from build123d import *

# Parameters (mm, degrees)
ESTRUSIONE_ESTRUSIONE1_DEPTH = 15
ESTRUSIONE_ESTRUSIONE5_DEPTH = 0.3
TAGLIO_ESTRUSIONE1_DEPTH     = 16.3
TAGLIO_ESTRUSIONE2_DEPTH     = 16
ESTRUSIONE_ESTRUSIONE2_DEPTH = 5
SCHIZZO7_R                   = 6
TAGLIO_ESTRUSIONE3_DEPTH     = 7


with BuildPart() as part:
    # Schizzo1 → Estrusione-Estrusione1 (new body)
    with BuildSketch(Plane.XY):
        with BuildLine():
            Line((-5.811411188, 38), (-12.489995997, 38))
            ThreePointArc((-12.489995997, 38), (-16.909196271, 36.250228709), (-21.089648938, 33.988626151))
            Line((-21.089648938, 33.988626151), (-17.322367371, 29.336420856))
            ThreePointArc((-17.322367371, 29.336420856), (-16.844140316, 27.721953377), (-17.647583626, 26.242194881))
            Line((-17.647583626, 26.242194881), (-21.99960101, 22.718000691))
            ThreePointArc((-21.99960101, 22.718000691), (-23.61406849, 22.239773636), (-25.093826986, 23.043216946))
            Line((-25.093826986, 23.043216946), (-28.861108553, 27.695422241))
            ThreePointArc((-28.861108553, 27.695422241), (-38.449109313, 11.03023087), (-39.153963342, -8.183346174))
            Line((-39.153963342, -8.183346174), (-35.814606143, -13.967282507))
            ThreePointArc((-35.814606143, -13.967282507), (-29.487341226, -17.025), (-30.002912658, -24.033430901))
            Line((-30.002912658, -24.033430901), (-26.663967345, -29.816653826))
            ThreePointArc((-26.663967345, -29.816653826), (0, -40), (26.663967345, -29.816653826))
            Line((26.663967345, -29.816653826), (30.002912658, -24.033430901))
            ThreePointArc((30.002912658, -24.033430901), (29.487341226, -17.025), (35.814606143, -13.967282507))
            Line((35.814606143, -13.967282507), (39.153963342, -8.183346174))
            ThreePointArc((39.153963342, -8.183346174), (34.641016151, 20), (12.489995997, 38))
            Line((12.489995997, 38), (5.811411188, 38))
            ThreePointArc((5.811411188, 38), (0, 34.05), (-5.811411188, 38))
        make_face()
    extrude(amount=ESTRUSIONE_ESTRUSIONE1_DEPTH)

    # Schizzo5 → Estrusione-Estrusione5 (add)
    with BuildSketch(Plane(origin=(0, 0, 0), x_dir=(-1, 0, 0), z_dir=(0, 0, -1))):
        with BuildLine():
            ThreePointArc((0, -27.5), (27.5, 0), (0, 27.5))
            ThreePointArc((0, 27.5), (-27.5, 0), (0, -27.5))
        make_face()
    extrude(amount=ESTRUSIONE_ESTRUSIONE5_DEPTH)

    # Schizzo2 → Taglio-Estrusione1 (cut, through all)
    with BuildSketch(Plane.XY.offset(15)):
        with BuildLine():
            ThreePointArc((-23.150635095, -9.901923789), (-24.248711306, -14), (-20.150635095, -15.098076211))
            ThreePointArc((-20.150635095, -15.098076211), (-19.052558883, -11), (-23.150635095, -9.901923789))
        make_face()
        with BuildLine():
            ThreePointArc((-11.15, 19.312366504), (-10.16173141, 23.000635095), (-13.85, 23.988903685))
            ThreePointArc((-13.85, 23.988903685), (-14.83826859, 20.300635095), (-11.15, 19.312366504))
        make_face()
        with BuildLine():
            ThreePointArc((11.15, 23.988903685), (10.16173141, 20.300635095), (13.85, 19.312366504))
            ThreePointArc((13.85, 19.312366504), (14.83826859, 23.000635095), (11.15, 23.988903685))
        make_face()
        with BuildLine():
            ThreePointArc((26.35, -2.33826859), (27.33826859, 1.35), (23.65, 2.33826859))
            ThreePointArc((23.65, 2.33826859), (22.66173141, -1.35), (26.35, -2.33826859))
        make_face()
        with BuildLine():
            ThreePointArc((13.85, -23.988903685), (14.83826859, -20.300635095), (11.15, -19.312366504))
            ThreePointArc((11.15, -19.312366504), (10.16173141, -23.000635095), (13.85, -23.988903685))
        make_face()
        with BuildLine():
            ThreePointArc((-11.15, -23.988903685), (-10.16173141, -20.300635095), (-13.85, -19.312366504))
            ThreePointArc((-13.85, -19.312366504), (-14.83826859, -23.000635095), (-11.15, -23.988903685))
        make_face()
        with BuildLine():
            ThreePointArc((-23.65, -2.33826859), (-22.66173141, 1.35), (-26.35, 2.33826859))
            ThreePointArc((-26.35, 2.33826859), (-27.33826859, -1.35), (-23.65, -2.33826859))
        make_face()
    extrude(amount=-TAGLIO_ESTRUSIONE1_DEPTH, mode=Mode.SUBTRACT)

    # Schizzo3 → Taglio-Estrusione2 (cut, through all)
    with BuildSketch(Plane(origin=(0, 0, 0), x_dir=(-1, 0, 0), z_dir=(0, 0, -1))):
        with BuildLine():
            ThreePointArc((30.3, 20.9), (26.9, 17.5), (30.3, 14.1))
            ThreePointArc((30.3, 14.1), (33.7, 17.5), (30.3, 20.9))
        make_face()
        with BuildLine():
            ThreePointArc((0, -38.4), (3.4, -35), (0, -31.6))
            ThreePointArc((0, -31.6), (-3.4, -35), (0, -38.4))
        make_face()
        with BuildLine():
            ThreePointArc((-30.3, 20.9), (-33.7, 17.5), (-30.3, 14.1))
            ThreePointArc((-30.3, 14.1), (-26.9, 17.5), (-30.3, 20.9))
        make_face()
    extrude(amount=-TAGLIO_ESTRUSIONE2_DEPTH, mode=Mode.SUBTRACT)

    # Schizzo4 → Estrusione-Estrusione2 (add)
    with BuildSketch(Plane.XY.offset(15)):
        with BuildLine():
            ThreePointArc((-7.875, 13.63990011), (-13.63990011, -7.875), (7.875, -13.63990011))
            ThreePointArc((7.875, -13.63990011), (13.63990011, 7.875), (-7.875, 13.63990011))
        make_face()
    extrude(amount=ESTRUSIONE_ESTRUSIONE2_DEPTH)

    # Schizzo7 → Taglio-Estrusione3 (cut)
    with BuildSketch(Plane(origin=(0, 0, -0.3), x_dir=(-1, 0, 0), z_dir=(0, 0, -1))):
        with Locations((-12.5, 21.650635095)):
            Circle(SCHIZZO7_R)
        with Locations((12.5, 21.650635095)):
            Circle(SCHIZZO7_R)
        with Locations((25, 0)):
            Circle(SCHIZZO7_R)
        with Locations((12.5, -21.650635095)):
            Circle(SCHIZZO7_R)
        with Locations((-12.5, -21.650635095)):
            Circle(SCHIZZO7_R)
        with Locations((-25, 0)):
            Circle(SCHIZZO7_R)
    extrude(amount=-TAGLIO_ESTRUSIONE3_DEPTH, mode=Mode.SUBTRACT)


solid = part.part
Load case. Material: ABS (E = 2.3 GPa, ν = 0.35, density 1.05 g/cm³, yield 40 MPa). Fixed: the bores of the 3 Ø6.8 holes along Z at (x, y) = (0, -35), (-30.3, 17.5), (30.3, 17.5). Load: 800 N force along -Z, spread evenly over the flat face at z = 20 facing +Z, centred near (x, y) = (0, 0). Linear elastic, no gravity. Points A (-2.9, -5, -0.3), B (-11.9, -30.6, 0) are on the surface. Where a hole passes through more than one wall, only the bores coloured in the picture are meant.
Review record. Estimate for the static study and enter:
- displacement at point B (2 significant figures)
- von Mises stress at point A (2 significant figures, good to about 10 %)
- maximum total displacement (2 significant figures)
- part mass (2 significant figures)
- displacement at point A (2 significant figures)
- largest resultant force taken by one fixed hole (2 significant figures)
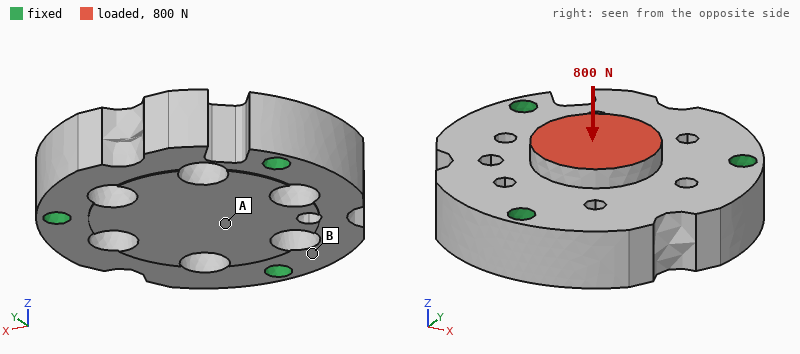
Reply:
12 µm
1.6 MPa
46 µm
71 g
41 µm
270 N
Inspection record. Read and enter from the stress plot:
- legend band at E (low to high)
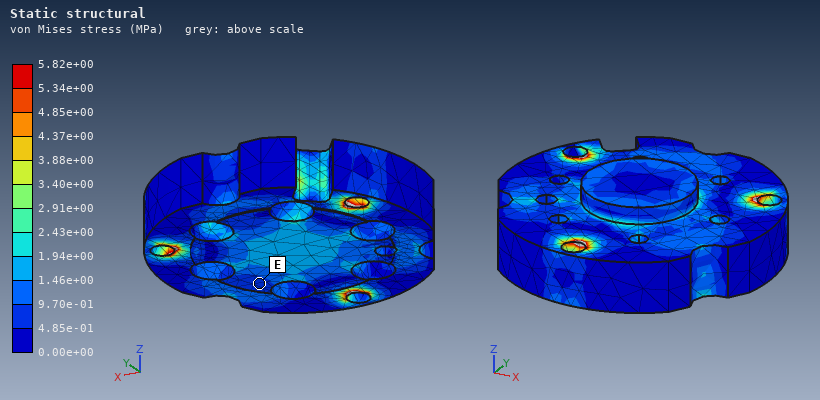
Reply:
4.85e-01 to 9.70e-01 MPa
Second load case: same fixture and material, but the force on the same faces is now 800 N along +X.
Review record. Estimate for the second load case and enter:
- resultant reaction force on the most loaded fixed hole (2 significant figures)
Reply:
360 N
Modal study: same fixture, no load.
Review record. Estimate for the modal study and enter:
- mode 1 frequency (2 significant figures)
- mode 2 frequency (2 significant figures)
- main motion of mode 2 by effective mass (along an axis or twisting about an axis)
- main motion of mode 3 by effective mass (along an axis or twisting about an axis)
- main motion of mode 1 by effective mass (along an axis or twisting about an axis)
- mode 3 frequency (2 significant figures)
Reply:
3300 Hz
3700 Hz
along Z
twisting about Y
along Z
4000 Hz
